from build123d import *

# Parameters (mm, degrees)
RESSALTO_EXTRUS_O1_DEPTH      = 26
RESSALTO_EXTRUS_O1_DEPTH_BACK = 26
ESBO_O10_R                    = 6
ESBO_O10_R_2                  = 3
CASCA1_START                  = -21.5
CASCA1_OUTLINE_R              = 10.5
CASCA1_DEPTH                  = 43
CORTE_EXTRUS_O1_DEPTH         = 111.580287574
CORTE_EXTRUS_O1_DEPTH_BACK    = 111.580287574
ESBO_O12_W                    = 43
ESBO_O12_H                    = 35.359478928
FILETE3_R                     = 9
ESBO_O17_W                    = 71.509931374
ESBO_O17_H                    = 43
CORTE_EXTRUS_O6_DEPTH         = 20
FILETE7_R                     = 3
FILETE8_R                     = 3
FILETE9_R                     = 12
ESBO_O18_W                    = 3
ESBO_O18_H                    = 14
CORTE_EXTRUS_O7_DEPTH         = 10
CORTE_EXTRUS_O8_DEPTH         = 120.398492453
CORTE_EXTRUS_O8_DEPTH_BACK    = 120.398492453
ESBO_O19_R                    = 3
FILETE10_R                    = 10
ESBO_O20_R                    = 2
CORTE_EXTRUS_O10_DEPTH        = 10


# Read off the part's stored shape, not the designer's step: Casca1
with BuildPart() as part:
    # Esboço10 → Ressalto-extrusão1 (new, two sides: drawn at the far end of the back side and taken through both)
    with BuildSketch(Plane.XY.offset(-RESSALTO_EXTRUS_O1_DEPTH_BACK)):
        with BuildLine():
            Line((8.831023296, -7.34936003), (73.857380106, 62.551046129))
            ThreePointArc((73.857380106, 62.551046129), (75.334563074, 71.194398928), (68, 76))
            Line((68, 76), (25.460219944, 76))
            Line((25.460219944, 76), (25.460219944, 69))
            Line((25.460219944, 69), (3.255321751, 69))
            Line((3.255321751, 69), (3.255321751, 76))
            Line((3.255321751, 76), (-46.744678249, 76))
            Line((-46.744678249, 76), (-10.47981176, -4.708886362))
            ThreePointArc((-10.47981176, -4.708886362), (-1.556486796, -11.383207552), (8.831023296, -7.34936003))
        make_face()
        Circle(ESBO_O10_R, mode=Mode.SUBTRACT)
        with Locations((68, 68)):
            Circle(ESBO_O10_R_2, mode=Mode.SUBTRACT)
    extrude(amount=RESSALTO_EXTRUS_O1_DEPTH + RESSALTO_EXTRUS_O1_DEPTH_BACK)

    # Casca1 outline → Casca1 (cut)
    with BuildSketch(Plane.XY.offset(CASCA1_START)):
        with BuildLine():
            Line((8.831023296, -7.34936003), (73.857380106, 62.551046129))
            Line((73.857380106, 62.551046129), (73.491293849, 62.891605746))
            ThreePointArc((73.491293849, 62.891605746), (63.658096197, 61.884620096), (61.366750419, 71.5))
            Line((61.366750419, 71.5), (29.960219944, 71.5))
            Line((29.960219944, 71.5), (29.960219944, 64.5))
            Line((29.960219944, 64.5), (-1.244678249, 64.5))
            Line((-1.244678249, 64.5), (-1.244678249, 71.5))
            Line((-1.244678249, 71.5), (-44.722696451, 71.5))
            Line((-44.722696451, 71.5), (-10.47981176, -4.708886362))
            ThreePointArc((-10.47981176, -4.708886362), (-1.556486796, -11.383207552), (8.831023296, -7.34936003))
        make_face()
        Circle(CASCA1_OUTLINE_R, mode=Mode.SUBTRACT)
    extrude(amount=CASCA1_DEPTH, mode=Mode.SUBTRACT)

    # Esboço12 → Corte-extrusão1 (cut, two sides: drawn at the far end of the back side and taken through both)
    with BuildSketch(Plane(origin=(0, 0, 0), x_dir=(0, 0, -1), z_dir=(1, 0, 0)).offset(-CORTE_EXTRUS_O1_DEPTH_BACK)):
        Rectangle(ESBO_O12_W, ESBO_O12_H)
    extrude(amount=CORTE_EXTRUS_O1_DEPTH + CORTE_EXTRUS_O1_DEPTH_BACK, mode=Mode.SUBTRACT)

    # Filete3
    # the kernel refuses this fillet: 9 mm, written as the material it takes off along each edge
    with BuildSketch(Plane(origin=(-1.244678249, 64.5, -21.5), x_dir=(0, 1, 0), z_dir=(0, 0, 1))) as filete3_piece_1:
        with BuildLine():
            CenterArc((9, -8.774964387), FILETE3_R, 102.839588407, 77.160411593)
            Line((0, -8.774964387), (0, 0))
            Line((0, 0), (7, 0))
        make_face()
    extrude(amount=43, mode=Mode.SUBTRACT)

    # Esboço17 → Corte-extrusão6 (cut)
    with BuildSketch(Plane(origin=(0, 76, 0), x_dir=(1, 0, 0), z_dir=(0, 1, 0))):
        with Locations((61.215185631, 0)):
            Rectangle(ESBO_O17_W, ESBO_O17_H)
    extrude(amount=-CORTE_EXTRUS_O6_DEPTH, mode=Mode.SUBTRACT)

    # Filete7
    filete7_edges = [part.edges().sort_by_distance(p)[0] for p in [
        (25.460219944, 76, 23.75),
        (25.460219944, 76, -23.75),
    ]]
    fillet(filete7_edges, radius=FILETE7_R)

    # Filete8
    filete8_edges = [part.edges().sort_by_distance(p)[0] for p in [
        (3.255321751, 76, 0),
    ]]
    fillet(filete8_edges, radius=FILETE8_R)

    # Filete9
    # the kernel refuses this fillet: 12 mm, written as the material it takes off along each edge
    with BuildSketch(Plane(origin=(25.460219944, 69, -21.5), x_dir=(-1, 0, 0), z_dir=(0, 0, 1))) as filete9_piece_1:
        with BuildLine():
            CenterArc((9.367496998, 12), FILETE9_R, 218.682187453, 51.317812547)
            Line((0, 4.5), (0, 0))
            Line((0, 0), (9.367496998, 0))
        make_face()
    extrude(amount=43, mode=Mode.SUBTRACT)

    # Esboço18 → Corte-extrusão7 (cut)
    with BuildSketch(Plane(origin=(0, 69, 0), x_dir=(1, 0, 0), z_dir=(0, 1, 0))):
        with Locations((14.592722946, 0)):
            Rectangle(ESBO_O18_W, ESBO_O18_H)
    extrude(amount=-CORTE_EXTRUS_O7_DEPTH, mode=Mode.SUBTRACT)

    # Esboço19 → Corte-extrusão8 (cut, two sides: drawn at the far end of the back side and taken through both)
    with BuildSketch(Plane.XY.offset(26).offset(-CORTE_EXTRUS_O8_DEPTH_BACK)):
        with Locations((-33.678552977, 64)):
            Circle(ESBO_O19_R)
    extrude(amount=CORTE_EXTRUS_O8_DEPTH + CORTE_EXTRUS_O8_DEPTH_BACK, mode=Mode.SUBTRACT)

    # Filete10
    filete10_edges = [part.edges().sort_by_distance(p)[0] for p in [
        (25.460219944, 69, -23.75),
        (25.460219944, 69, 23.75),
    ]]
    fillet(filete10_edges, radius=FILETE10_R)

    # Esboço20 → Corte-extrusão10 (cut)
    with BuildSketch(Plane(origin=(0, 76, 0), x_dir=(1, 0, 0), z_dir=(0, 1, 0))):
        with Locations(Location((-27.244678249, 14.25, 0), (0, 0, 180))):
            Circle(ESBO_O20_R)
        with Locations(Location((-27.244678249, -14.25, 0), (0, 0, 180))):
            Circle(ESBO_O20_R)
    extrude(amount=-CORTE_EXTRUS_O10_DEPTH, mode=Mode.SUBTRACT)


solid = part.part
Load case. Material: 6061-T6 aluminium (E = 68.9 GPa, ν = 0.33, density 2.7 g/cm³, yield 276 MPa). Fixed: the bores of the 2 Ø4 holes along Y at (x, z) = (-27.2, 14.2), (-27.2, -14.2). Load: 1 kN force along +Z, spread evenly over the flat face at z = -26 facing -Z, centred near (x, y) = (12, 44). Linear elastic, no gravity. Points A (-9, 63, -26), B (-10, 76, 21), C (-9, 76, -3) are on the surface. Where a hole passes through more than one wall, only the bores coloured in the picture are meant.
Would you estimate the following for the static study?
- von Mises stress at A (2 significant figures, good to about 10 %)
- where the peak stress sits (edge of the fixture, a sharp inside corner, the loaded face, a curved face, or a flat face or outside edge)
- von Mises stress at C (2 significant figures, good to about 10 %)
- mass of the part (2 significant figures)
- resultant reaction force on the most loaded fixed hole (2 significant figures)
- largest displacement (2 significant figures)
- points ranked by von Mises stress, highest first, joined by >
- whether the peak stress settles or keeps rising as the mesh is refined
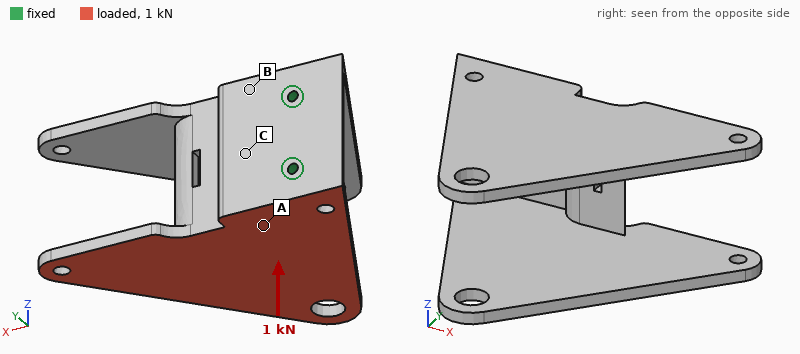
76 MPa
edge of the fixture
42 MPa
180 g
1.6 kN
1.8 mm
A > C > B
keeps rising
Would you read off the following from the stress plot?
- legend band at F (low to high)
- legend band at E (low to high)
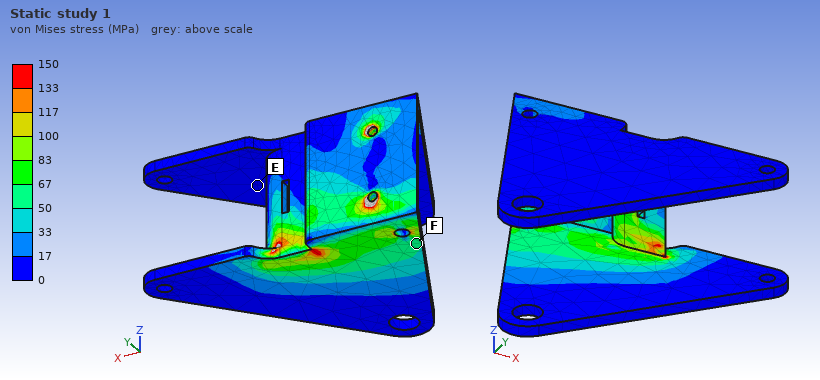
50 to 67 MPa
0 to 17 MPa
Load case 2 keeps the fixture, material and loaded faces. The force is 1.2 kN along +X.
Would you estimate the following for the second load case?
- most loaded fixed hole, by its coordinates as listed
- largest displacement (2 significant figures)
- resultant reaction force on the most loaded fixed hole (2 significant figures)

(-27.2, -14.2)
1.0 mm
1.6 kN
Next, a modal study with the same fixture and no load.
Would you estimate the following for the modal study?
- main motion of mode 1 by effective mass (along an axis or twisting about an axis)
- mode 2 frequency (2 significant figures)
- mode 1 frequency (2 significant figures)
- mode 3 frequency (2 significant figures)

along Z
520 Hz
490 Hz
650 Hz
